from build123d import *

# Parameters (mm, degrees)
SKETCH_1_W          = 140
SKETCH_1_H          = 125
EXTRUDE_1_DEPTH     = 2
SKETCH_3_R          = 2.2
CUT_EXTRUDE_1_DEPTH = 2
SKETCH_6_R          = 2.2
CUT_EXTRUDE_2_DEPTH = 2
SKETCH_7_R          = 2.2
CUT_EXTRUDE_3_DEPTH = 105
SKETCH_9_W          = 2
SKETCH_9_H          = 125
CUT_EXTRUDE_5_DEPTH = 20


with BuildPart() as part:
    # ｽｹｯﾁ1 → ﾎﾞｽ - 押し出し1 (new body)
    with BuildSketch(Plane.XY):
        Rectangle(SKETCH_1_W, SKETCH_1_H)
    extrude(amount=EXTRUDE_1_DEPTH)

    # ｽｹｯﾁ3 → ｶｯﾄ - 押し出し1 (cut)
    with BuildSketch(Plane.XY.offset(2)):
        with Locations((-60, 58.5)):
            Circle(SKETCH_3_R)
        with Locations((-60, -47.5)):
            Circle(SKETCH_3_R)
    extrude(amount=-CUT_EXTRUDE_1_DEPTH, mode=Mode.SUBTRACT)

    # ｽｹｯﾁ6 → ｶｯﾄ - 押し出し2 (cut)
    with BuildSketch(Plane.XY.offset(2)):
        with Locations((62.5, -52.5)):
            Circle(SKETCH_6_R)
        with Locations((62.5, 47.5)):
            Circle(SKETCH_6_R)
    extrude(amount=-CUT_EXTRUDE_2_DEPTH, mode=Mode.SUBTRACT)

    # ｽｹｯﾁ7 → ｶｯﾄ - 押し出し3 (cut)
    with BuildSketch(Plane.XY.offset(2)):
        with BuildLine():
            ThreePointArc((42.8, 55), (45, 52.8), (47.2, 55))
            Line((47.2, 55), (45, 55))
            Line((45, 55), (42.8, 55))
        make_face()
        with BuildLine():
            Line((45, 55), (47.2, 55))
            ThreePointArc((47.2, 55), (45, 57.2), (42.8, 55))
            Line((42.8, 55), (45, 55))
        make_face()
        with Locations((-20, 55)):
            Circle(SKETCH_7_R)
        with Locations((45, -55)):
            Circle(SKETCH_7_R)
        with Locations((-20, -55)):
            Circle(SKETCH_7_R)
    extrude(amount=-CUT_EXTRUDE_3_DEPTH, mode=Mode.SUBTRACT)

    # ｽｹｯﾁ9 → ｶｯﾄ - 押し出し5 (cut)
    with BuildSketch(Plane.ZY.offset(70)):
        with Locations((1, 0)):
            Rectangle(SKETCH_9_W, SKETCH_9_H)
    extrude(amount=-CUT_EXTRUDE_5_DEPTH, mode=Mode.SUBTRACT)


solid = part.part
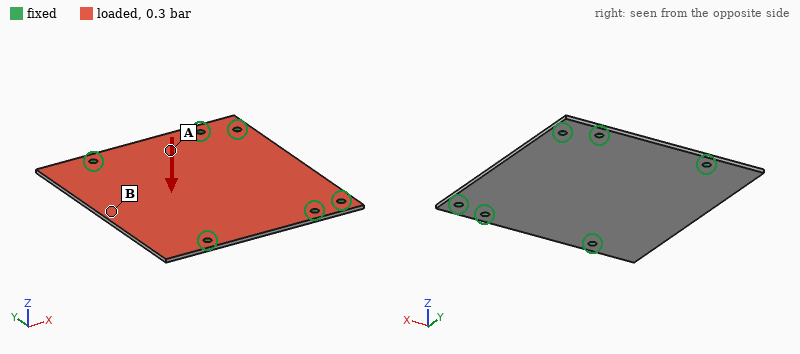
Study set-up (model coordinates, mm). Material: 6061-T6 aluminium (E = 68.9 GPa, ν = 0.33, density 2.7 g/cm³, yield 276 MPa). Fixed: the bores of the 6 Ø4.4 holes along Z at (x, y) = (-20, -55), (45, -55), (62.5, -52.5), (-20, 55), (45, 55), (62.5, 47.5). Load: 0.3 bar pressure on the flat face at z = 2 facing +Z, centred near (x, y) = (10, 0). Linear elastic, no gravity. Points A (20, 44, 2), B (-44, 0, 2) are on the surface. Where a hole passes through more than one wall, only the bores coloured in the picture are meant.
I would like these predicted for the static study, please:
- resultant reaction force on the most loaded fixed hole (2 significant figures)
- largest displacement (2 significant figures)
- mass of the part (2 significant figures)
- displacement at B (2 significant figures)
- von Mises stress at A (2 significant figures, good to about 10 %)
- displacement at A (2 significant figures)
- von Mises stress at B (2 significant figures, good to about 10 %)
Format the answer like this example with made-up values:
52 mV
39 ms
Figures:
120 N
0.43 mm
81 g
0.40 mm
12 MPa
0.086 mm
26 MPa
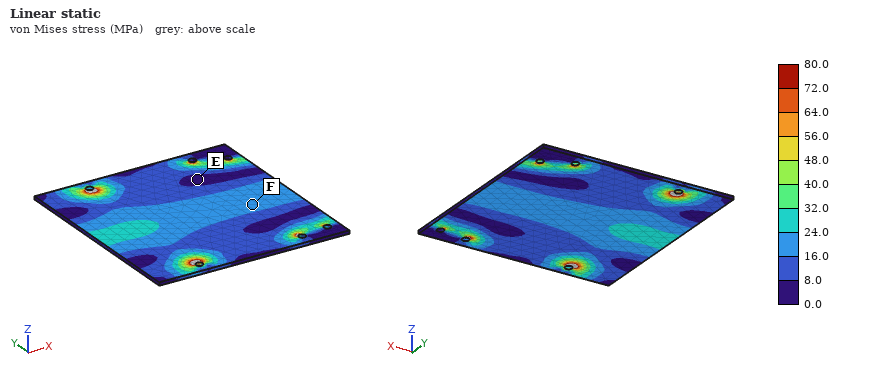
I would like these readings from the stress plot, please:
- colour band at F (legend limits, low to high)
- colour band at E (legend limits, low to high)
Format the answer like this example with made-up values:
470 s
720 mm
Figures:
16.0 to 24.0 MPa
0.0 to 8.0 MPa
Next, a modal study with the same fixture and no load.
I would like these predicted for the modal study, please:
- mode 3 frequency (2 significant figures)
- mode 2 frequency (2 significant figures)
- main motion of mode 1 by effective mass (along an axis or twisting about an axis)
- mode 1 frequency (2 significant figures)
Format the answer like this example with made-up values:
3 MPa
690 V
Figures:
1400 Hz
960 Hz
along Z
740 Hz
